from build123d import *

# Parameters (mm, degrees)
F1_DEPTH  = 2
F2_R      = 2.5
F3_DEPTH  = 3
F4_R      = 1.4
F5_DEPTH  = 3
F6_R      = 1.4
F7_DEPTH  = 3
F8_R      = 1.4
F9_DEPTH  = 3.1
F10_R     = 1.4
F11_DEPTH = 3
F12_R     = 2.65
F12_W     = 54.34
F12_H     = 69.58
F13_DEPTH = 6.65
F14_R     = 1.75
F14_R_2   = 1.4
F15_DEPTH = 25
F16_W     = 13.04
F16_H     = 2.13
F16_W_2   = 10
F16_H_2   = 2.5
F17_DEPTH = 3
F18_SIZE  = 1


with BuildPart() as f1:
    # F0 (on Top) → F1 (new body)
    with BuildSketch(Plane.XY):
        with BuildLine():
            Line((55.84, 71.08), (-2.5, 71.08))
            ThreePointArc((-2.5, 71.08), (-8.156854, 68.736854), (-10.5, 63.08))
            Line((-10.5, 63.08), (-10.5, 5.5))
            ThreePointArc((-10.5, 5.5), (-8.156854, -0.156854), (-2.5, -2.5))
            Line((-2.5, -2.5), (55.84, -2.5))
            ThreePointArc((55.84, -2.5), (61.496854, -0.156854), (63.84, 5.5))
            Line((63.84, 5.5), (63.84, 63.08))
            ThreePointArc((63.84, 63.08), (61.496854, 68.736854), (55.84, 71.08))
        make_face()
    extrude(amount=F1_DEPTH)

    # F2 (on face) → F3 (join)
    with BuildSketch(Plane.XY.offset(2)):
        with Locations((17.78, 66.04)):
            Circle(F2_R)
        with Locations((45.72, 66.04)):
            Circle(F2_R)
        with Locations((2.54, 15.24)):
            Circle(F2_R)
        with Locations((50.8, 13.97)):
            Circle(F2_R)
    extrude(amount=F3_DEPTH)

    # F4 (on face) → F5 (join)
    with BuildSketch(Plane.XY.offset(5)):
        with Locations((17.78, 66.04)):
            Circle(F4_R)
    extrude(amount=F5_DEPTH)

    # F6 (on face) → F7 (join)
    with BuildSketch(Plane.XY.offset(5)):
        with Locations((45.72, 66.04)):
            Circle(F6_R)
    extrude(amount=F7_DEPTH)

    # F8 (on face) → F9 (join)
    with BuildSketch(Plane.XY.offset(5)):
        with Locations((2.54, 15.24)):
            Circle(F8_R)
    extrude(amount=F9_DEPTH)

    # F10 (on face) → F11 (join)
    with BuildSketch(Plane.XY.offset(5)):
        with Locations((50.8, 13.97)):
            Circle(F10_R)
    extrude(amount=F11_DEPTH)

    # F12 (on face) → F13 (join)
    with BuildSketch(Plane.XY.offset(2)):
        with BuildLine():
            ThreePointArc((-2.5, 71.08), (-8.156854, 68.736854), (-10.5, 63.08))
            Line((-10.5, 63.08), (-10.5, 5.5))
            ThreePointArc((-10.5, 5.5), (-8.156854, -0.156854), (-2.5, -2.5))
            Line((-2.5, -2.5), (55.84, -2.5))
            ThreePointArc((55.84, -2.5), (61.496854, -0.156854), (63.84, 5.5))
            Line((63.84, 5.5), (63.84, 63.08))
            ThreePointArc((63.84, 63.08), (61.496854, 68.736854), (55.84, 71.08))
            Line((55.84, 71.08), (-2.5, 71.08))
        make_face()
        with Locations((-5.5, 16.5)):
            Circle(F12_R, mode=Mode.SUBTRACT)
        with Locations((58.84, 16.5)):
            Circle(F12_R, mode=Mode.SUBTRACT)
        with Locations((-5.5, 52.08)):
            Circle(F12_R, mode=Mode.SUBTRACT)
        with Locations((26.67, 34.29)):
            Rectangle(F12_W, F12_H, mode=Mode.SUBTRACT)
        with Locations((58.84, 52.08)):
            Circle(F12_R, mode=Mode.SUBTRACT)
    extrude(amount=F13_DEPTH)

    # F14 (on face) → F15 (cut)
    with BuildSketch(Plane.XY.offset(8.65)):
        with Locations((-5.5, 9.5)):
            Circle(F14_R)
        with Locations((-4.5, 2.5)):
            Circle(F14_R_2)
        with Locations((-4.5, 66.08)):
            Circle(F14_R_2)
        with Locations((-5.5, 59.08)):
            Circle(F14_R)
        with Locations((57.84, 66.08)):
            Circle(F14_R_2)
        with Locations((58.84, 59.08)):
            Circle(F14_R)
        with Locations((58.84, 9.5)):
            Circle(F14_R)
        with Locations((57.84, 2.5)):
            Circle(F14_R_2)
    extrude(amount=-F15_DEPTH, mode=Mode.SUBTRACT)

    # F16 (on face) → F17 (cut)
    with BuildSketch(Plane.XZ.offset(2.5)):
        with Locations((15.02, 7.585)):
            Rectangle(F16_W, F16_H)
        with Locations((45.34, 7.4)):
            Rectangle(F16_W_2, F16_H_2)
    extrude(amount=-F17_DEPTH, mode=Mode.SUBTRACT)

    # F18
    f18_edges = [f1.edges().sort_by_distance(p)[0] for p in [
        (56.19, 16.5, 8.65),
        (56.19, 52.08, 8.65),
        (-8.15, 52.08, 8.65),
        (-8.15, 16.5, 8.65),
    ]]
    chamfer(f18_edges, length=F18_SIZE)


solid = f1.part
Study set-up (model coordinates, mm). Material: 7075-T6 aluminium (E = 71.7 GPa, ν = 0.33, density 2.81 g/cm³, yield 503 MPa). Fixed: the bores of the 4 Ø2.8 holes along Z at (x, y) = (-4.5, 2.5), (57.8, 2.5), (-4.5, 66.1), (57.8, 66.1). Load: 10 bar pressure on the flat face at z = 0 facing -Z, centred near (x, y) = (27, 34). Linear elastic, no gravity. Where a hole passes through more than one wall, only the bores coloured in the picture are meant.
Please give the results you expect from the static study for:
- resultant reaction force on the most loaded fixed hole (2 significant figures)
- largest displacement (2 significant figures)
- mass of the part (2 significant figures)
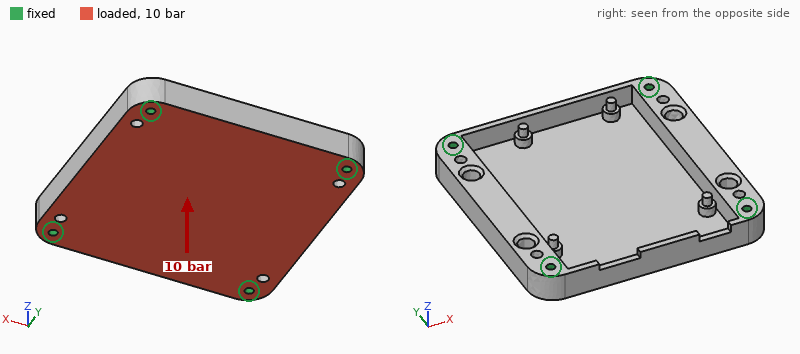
1.6 kN
0.52 mm
58 g
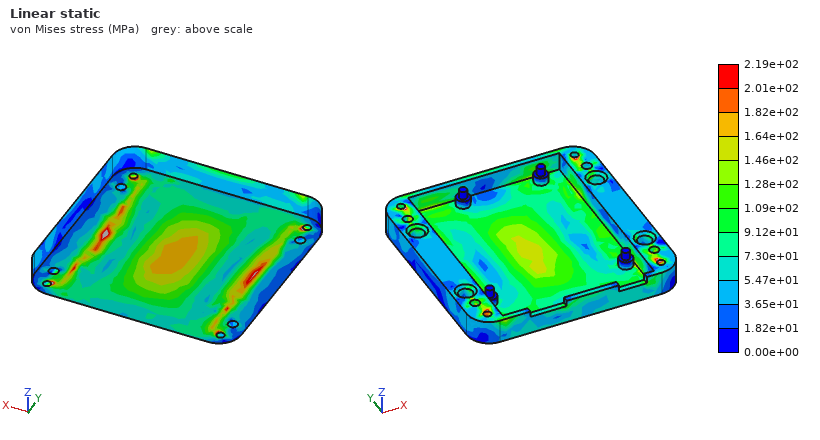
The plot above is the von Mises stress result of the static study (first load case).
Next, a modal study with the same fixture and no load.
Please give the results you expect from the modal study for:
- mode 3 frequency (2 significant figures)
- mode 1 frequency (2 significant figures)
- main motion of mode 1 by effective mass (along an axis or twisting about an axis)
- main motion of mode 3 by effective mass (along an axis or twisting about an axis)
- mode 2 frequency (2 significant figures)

7600 Hz
3700 Hz
along Z
twisting about Y
5900 Hz
